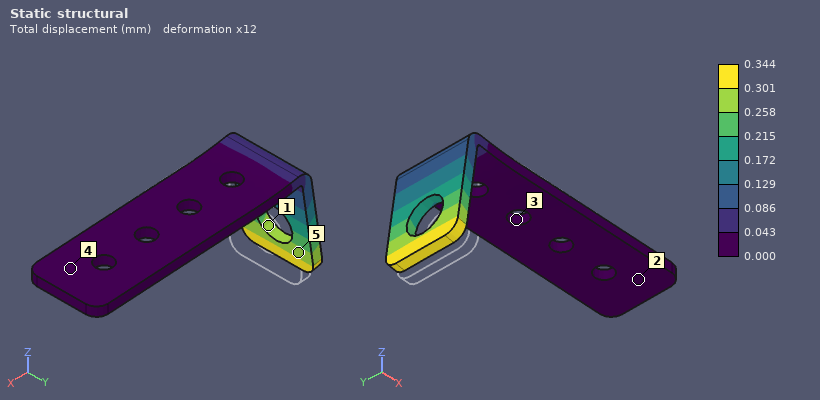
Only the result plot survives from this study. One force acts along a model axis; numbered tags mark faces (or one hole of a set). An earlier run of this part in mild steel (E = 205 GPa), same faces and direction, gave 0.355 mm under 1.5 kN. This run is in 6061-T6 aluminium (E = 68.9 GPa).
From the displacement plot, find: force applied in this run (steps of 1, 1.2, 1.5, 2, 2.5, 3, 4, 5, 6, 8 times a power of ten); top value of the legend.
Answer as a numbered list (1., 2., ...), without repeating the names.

1. 500 N
2. 0.344 mm
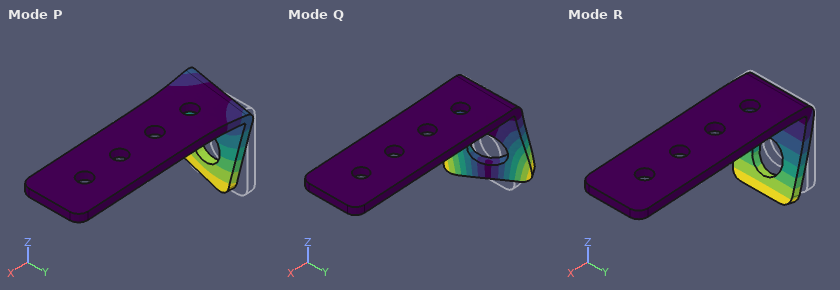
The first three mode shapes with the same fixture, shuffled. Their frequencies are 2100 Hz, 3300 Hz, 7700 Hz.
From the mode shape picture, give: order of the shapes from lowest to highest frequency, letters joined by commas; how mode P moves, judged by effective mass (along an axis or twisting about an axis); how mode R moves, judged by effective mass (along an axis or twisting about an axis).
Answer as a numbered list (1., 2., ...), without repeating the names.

1. R, P, Q
2. along Y
3. along X
